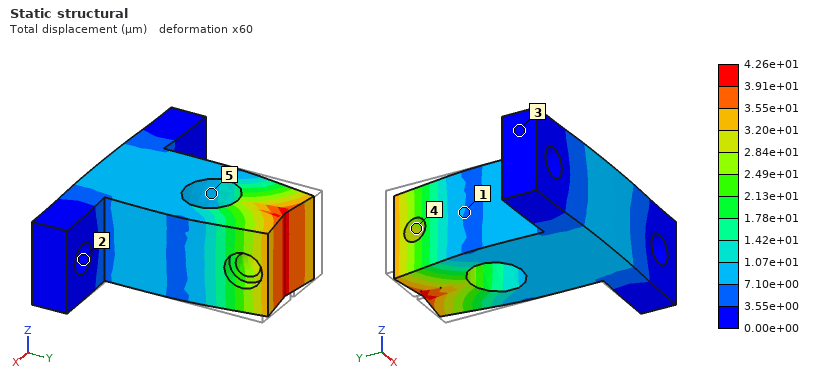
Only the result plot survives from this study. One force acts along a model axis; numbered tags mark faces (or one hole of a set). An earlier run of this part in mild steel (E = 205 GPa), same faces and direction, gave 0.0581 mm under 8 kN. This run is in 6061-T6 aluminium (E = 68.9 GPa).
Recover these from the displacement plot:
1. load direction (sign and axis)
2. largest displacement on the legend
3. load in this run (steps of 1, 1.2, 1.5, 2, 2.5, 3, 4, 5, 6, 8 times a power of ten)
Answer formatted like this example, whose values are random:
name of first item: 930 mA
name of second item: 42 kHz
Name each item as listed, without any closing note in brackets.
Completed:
load direction: -Y
largest displacement on the legend: 4.26e+01 µm
load in this run: 2 kN
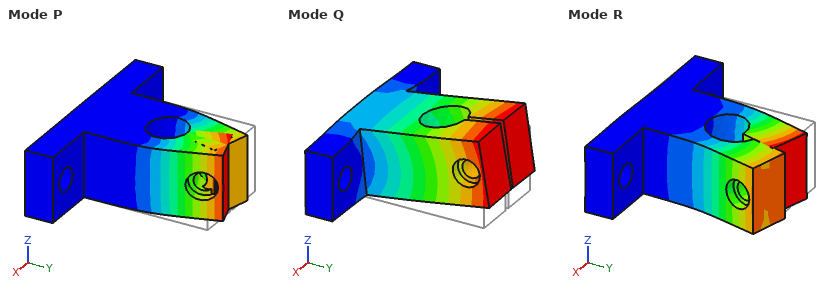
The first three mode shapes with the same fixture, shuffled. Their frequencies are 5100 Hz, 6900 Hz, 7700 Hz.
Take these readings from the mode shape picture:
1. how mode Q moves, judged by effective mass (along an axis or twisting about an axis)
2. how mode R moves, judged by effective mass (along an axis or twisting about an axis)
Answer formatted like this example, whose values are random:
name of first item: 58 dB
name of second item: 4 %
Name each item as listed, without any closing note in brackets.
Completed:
how mode Q moves, judged by effective mass: along Z
how mode R moves, judged by effective mass: along X
